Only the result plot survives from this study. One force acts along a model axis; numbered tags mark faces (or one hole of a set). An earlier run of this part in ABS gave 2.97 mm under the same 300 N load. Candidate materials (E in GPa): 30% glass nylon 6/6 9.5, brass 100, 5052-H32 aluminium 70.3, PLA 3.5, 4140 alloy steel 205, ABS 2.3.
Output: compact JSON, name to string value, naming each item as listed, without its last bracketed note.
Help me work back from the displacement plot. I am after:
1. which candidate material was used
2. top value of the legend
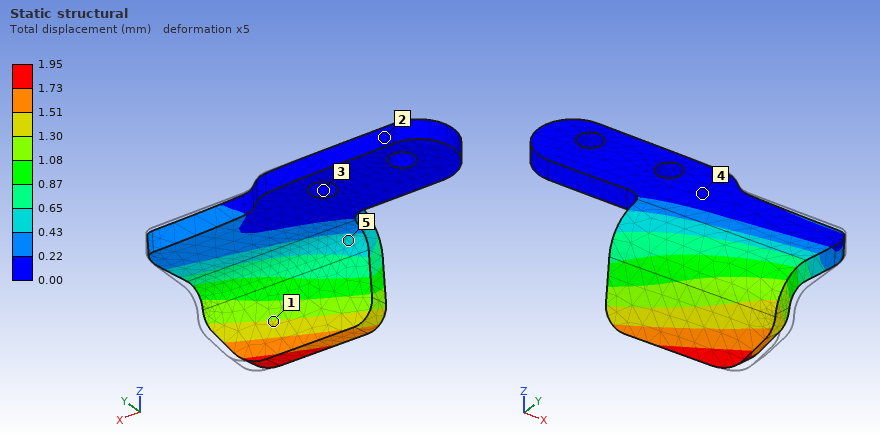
{"which candidate material was used": "PLA", "top value of the legend": "1.95 mm"}
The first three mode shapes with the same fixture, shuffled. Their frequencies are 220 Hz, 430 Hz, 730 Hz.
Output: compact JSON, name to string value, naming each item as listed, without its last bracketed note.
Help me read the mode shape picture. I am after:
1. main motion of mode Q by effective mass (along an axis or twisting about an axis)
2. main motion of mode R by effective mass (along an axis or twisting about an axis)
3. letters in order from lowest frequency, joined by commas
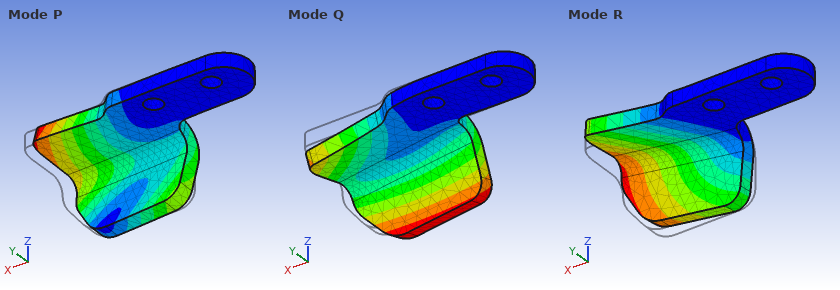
{"main motion of mode Q by effective mass": "along Y", "main motion of mode R by effective mass": "along Z", "letters in order from lowest frequency, joined by commas": "R, Q, P"}
